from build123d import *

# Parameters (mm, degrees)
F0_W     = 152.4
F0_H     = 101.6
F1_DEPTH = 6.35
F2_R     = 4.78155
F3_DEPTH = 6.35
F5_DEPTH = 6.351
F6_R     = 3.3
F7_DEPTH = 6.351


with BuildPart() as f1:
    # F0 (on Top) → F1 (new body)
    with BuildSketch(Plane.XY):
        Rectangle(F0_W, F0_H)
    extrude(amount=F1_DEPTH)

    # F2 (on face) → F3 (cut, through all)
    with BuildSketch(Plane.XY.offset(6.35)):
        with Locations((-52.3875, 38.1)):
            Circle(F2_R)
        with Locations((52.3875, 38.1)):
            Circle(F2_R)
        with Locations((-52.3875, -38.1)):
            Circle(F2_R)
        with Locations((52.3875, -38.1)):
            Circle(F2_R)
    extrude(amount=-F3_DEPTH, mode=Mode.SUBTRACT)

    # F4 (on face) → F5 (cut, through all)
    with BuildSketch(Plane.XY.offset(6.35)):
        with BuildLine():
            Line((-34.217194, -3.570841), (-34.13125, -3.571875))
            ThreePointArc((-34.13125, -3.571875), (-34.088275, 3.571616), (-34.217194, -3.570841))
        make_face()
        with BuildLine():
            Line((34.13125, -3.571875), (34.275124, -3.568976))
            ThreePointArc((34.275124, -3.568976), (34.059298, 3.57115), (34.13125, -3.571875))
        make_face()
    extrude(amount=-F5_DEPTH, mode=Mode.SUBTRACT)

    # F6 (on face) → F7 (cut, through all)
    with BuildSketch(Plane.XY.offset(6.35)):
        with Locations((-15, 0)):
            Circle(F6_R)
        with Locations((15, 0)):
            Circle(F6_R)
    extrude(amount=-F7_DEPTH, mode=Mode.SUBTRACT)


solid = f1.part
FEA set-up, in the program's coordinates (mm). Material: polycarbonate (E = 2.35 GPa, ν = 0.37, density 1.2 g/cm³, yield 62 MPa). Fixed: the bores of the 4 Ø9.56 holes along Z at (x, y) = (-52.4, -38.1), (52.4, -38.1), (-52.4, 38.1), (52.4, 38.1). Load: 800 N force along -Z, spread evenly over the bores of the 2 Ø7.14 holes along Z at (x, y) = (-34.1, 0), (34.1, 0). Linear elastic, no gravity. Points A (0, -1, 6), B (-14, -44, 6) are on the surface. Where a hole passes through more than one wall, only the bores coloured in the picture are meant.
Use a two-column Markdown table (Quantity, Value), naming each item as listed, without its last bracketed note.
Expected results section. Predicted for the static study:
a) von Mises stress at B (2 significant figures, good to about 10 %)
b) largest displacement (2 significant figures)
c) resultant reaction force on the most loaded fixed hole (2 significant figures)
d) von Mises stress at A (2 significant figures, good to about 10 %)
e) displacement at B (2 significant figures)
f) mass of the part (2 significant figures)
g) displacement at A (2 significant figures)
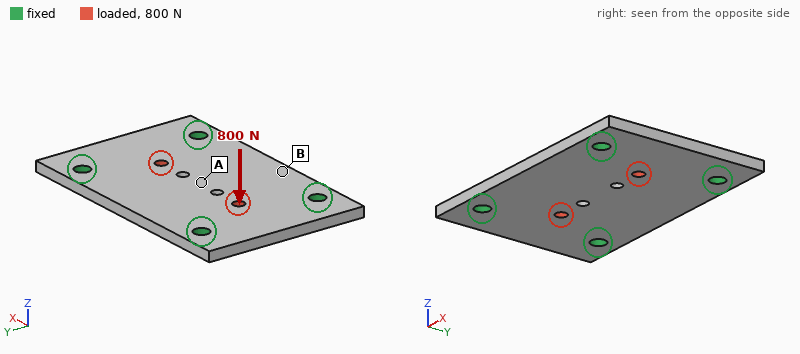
| Quantity | Value |
|---|---|
| von Mises stress at B | 2.2 MPa |
| largest displacement | 0.71 mm |
| resultant reaction force on the most loaded fixed hole | 200 N |
| von Mises stress at A | 6.5 MPa |
| displacement at B | 0.19 mm |
| mass of the part | 110 g |
| displacement at A | 0.70 mm |
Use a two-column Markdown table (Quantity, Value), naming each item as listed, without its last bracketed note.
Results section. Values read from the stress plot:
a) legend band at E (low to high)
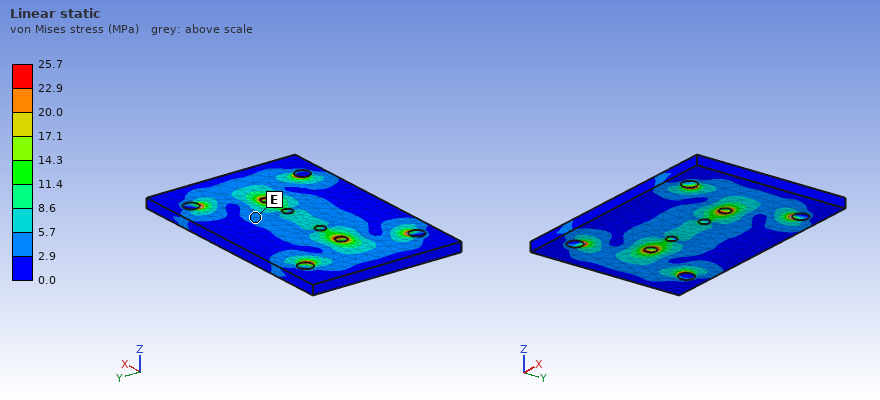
| Quantity | Value |
|---|---|
| legend band at E | 2.9 to 5.7 MPa |
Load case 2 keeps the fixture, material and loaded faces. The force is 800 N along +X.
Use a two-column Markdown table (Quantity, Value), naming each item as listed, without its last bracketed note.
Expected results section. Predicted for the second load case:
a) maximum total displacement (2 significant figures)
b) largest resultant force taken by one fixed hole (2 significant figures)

| Quantity | Value |
|---|---|
| maximum total displacement | 33 µm |
| largest resultant force taken by one fixed hole | 210 N |
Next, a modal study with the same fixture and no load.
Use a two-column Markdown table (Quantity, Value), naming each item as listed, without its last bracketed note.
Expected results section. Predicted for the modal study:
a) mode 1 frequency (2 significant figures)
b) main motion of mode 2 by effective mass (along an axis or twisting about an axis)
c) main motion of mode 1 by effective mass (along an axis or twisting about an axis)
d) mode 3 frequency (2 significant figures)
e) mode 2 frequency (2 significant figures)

| Quantity | Value |
|---|---|
| mode 1 frequency | 770 Hz |
| main motion of mode 2 by effective mass | twisting about X |
| main motion of mode 1 by effective mass | along Z |
| mode 3 frequency | 1400 Hz |
| mode 2 frequency | 1100 Hz |
